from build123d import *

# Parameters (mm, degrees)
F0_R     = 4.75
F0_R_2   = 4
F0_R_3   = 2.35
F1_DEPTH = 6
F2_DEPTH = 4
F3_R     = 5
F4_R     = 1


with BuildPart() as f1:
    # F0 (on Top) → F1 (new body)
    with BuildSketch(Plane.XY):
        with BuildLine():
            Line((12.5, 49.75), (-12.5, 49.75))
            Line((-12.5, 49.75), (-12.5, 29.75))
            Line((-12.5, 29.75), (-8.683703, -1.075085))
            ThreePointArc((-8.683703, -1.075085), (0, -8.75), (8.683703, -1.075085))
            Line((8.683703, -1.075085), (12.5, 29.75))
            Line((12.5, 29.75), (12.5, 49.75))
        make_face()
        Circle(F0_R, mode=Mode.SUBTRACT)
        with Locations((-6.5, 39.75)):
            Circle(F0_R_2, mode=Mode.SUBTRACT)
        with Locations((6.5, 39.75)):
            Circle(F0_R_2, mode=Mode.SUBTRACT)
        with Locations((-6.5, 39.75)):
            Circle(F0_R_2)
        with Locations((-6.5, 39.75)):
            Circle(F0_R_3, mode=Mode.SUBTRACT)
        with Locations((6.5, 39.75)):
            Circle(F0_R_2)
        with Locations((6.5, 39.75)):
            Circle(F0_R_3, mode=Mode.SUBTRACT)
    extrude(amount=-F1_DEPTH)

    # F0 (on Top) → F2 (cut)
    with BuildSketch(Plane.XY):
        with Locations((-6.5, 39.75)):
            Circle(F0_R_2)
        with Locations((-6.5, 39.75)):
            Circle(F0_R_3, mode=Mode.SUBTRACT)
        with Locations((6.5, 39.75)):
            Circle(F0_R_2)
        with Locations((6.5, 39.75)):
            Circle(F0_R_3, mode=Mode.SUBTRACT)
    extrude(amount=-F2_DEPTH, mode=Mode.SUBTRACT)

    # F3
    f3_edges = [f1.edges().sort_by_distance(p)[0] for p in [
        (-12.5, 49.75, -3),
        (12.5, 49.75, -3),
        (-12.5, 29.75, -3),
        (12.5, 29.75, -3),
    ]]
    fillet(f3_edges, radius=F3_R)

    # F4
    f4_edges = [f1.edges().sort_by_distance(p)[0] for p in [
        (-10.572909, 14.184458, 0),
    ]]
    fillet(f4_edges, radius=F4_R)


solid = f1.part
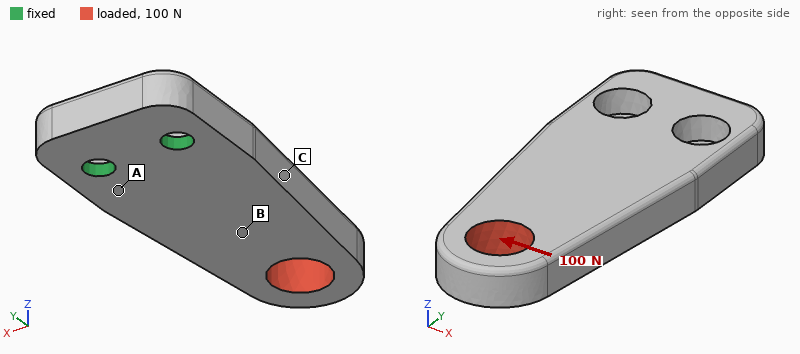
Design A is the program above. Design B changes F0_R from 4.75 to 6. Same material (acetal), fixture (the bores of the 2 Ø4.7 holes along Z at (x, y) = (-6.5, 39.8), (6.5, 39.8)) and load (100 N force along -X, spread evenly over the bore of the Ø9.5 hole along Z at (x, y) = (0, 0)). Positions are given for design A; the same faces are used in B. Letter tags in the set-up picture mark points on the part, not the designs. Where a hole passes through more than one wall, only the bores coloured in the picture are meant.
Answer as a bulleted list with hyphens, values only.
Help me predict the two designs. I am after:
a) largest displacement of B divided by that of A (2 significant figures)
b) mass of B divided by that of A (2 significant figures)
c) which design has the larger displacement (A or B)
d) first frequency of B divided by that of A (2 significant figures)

- 1.1
- 0.96
- B
- 1.1
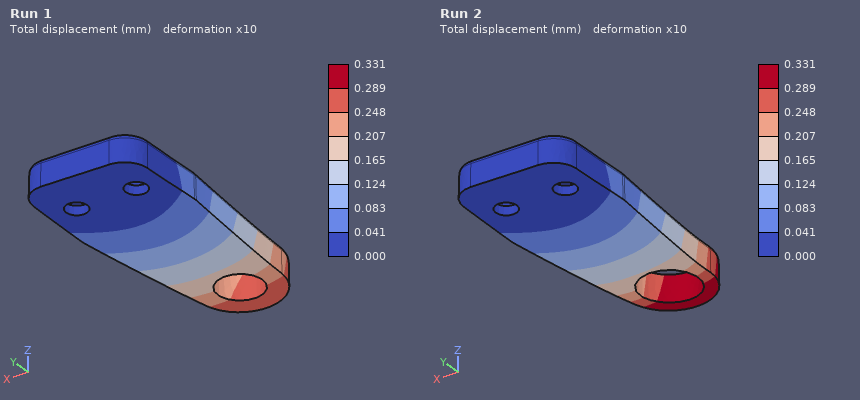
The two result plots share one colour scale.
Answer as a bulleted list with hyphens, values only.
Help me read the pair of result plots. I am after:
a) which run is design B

- Run 2
